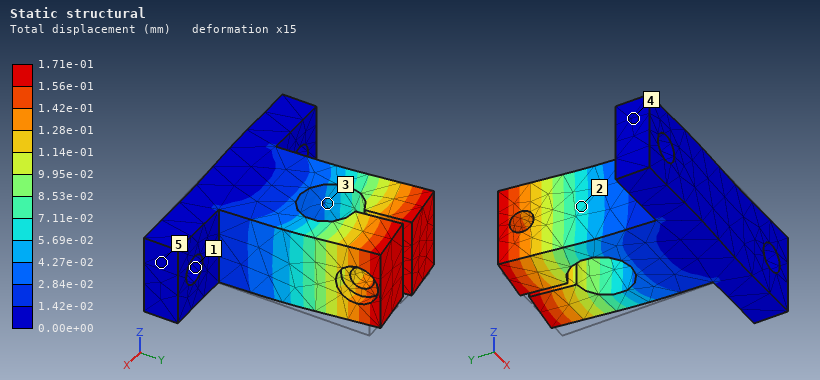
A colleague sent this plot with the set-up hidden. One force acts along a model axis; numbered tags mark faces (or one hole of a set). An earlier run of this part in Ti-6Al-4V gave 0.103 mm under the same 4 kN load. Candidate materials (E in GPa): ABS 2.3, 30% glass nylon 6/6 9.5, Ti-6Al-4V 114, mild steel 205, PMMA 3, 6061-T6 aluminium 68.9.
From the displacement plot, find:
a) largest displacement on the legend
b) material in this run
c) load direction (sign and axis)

1.71e-01 mm
6061-T6 aluminium
-X
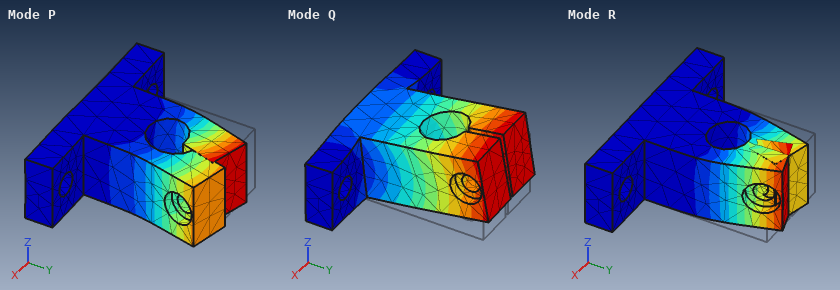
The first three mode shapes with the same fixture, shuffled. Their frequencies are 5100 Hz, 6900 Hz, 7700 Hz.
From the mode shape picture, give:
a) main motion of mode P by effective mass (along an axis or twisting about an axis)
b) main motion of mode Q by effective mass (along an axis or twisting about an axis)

along X
along Z
